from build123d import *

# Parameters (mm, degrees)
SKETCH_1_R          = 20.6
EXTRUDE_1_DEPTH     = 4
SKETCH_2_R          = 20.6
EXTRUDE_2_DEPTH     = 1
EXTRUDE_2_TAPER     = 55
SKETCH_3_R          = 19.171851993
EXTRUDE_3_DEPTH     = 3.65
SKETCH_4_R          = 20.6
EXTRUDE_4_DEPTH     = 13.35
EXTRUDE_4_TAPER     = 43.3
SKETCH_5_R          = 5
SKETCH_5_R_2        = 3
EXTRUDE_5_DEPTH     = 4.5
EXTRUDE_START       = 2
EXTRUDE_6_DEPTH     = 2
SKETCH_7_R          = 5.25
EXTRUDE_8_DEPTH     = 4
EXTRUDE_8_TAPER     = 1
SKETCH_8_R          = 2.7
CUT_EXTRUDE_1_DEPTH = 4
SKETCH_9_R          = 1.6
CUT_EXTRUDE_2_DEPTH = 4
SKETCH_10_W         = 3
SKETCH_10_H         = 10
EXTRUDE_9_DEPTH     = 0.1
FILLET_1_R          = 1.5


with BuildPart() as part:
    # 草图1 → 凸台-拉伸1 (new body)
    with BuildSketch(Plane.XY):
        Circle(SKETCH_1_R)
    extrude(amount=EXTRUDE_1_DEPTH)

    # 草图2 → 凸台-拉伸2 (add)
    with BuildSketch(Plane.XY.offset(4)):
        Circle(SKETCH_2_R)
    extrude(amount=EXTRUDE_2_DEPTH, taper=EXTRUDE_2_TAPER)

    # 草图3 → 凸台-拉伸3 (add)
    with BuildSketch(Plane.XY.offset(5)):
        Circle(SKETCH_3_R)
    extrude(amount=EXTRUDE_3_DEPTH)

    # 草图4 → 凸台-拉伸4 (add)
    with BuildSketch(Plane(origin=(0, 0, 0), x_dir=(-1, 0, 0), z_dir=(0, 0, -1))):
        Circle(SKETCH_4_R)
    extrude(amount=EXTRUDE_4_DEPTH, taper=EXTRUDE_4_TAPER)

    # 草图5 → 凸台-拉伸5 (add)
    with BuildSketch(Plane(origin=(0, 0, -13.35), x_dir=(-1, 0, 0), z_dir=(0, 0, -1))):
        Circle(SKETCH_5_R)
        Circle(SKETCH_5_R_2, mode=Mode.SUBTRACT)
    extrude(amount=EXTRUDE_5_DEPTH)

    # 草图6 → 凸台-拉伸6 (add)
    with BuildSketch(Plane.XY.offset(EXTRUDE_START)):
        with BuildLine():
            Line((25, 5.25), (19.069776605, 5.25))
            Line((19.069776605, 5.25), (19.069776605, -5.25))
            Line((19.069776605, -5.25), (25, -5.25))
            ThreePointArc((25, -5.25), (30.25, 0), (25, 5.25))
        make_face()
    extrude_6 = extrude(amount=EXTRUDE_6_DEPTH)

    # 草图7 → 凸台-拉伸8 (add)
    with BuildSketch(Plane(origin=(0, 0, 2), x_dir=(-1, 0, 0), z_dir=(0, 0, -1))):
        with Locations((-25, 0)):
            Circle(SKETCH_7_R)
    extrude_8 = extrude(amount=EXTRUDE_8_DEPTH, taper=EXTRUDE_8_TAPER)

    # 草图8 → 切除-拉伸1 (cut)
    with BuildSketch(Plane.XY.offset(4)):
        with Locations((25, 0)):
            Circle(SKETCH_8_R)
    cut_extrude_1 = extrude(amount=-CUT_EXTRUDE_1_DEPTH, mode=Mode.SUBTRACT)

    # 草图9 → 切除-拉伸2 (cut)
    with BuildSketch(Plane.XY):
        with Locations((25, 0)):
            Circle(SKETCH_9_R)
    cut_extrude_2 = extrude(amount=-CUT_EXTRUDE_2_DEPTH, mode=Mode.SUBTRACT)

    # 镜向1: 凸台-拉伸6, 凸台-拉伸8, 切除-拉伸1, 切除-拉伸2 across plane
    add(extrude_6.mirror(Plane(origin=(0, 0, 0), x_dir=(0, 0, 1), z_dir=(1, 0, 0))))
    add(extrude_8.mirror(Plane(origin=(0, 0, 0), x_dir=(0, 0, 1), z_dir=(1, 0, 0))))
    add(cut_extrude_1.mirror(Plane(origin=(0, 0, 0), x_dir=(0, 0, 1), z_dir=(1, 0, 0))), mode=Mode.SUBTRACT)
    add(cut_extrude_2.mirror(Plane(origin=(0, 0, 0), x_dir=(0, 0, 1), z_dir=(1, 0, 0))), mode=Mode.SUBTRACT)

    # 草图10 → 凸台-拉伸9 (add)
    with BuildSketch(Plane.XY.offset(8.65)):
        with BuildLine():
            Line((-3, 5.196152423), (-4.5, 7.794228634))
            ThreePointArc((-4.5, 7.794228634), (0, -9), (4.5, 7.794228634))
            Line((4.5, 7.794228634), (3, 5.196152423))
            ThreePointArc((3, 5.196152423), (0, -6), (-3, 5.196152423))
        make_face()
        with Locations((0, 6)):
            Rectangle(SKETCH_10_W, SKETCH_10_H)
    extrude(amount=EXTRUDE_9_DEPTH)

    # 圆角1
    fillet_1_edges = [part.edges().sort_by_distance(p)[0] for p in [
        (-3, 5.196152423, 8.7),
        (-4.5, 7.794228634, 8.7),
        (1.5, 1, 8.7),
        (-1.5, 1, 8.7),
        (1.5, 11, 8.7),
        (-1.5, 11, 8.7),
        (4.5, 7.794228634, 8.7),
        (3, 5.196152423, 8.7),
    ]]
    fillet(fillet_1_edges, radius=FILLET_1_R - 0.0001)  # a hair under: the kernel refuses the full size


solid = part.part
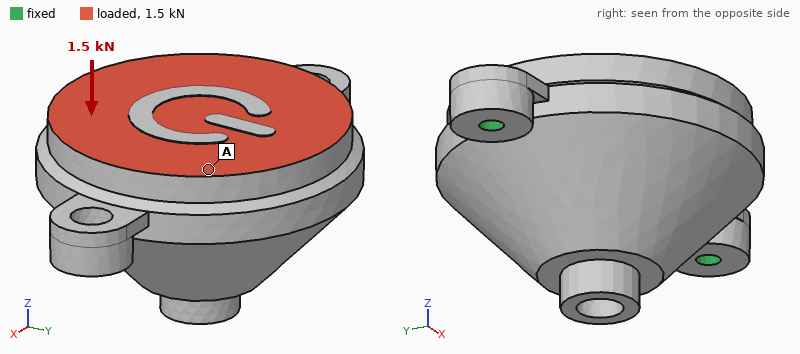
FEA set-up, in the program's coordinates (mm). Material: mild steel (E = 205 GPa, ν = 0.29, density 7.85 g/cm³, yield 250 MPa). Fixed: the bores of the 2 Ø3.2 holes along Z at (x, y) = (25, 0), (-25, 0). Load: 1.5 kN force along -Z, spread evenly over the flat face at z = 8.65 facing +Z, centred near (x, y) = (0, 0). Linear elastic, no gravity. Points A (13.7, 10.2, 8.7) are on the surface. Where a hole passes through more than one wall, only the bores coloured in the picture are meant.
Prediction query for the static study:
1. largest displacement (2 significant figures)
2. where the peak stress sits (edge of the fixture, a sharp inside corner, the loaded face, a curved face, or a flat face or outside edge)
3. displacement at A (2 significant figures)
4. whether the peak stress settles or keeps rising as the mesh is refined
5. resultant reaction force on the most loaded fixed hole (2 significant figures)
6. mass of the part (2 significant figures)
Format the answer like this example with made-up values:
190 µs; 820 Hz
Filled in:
5.0 µm; edge of the fixture; 4.4 µm; keeps rising; 920 N; 160 g
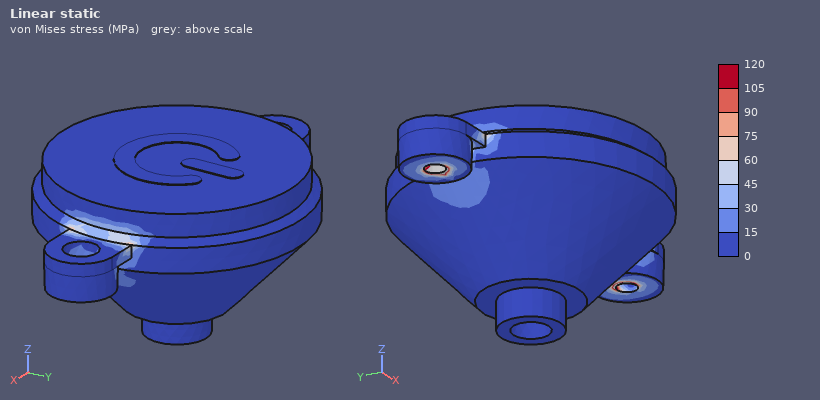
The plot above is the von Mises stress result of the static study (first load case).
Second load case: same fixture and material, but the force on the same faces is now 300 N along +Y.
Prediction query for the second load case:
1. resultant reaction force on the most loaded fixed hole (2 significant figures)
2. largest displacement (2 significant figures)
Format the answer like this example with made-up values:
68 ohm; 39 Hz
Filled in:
150 N; 17 µm
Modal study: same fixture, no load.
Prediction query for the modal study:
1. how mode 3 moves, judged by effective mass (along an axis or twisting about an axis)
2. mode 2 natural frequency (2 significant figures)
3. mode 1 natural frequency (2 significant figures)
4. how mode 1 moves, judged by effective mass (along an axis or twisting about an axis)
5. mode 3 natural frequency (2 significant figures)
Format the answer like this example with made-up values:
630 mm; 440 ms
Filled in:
along Y; 7300 Hz; 2200 Hz; twisting about X; 7600 Hz
